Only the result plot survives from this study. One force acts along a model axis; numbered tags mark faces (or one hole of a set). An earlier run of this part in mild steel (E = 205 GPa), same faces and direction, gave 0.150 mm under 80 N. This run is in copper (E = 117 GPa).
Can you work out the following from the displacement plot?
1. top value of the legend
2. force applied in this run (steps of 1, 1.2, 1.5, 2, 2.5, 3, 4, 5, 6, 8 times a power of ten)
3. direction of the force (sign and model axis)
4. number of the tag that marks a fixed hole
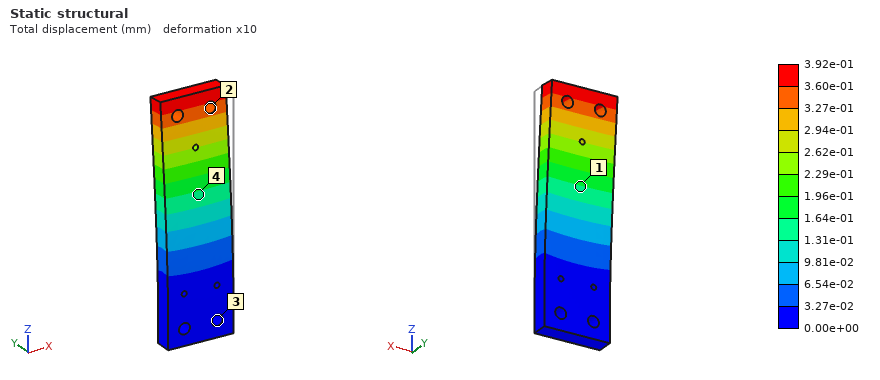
3.92e-01 mm
120 N
+Y
3
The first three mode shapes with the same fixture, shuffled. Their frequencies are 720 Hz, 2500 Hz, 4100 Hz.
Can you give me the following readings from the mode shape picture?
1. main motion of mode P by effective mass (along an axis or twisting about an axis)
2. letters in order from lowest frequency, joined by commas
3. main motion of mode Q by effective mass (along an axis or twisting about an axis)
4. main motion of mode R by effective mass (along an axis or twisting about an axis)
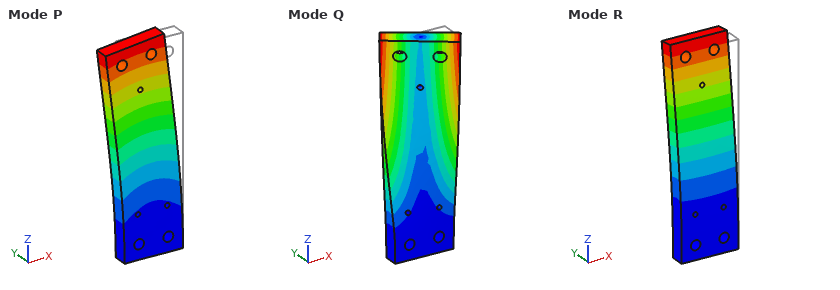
along X
R, P, Q
twisting about Z
along Y
